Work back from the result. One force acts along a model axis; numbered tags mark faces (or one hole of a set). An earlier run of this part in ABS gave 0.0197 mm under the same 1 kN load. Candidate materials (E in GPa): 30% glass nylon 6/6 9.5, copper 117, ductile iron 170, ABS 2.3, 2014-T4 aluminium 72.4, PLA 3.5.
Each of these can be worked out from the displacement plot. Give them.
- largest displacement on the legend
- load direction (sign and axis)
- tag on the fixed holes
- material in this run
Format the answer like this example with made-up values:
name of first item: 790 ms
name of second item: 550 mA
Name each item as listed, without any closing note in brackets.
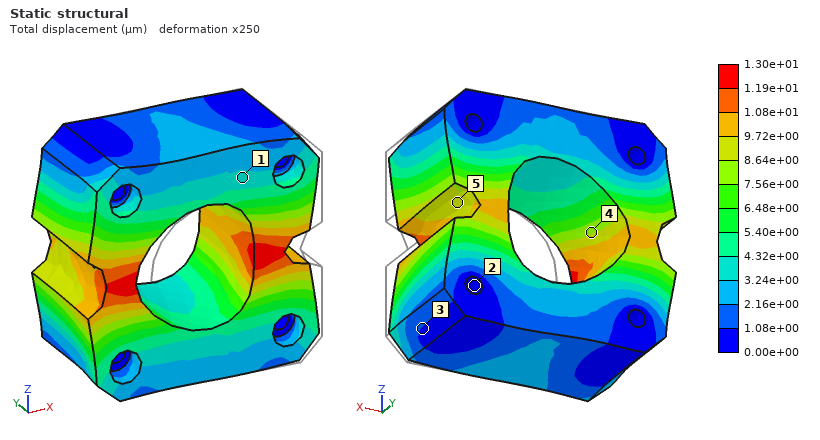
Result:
largest displacement on the legend: 1.30e+01 µm
load direction: -X
tag on the fixed holes: 2
material in this run: PLA
